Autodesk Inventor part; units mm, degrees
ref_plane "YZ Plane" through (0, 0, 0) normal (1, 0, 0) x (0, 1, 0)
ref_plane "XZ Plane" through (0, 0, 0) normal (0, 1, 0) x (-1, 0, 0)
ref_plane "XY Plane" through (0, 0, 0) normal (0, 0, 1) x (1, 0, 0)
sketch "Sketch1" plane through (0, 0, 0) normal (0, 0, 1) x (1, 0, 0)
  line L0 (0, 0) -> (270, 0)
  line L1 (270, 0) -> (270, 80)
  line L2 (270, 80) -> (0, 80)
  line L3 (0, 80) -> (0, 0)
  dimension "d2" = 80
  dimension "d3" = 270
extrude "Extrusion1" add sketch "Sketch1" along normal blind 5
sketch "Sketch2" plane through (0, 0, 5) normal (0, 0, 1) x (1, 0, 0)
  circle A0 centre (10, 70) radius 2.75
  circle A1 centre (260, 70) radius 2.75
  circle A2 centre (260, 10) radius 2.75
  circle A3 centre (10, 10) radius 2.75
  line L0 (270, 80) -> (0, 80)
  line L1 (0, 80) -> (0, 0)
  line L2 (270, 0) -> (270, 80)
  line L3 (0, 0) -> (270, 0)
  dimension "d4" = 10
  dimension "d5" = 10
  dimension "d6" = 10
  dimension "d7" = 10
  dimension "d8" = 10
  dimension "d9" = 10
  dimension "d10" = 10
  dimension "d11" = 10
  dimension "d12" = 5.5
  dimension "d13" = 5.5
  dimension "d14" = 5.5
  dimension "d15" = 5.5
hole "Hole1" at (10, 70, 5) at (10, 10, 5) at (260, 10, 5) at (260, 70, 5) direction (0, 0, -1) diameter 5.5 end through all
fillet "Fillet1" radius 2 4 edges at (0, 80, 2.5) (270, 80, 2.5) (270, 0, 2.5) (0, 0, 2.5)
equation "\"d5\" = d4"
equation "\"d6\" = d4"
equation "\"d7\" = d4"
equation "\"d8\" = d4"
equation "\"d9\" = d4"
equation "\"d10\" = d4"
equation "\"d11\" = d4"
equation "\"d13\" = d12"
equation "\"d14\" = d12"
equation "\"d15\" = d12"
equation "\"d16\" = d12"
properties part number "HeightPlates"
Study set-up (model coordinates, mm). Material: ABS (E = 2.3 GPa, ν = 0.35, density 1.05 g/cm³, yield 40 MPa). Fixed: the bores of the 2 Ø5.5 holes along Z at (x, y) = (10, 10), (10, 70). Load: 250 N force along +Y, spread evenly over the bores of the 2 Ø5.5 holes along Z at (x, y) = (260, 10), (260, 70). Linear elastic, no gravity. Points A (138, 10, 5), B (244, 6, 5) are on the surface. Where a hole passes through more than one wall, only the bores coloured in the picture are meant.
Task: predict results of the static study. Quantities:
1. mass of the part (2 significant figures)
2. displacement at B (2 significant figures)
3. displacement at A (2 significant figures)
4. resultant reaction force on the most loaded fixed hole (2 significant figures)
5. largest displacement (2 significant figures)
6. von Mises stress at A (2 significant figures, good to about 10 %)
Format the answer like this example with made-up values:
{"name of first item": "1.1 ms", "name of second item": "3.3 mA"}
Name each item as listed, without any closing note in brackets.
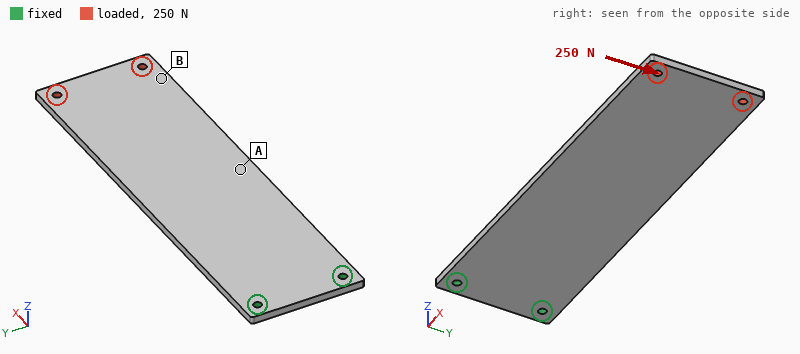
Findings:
{"mass of the part": "110 g", "displacement at B": "2.8 mm", "displacement at A": "1.1 mm", "resultant reaction force on the most loaded fixed hole": "1.0 kN", "largest displacement": "3.2 mm", "von Mises stress at A": "4.4 MPa"}
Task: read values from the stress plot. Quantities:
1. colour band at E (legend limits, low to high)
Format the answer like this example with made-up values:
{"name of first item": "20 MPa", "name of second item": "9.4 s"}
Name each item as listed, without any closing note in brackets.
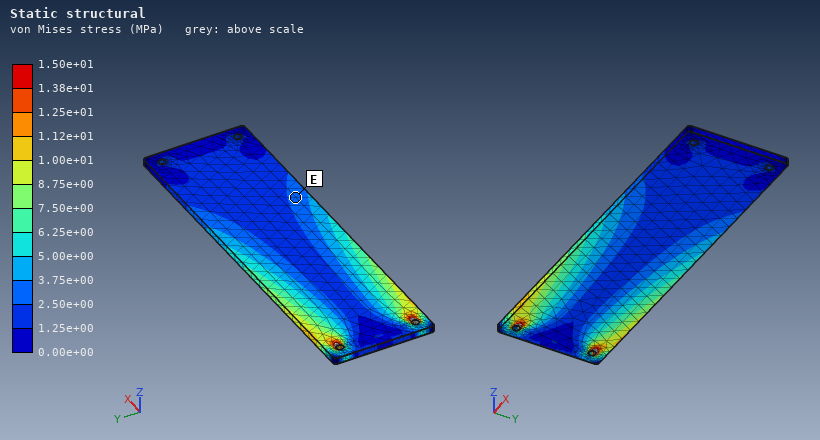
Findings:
{"colour band at E": "2.50e+00 to 3.75e+00 MPa"}
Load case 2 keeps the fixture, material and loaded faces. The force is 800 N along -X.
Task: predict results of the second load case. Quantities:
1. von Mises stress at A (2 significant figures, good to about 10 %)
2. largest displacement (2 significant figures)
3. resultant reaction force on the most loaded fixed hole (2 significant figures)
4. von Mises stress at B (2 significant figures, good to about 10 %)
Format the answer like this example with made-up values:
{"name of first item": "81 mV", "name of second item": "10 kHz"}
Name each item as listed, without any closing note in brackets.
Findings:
{"von Mises stress at A": "2.0 MPa", "largest displacement": "0.27 mm", "resultant reaction force on the most loaded fixed hole": "410 N", "von Mises stress at B": "3.2 MPa"}
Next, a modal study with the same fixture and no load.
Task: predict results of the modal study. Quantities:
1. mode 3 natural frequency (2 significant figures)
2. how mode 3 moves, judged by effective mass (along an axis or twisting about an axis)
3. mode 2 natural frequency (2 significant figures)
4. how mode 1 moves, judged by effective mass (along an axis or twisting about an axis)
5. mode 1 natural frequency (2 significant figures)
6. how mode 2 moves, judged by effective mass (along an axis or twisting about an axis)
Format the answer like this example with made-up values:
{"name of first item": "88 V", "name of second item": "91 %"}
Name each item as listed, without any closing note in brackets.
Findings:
{"mode 3 natural frequency": "120 Hz", "how mode 3 moves, judged by effective mass": "twisting about X", "mode 2 natural frequency": "110 Hz", "how mode 1 moves, judged by effective mass": "along Z", "mode 1 natural frequency": "17 Hz", "how mode 2 moves, judged by effective mass": "along Z"}
